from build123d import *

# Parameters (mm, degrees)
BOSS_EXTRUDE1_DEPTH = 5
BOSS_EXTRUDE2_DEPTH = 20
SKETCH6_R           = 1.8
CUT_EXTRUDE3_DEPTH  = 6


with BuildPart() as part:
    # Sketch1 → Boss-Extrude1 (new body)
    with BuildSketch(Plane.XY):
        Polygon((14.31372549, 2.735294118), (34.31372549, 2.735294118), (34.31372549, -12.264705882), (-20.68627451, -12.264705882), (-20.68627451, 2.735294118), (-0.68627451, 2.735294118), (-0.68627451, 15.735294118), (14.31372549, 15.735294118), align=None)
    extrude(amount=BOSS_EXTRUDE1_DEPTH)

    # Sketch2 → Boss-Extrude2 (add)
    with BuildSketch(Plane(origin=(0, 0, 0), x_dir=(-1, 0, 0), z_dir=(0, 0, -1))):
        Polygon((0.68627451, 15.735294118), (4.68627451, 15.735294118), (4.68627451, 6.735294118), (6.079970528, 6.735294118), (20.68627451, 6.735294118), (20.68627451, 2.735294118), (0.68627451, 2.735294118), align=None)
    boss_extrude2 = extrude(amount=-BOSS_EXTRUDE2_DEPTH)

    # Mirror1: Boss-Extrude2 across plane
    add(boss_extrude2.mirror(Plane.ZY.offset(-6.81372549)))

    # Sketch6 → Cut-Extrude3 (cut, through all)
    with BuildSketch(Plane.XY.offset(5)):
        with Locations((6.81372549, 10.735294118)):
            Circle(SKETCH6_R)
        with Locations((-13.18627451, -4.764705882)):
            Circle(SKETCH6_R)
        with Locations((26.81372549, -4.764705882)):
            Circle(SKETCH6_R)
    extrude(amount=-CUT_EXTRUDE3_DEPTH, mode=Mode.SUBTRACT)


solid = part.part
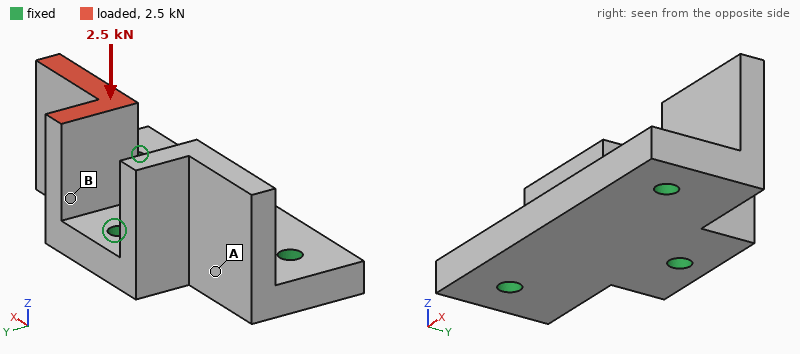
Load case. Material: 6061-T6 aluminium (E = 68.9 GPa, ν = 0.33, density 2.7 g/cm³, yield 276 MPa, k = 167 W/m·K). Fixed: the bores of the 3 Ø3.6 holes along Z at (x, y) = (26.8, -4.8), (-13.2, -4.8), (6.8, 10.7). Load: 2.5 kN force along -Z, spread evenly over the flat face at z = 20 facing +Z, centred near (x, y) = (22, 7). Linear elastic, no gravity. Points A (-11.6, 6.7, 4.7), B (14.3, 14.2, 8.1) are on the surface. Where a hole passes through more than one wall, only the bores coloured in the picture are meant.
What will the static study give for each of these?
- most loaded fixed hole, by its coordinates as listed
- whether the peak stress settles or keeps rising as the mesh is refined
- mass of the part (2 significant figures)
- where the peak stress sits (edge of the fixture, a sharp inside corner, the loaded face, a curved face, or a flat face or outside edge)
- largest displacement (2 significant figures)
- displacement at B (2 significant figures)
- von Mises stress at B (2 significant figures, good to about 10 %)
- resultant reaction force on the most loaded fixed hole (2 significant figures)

(26.8, -4.8)
keeps rising
26 g
edge of the fixture
75 µm
32 µm
54 MPa
1.4 kN
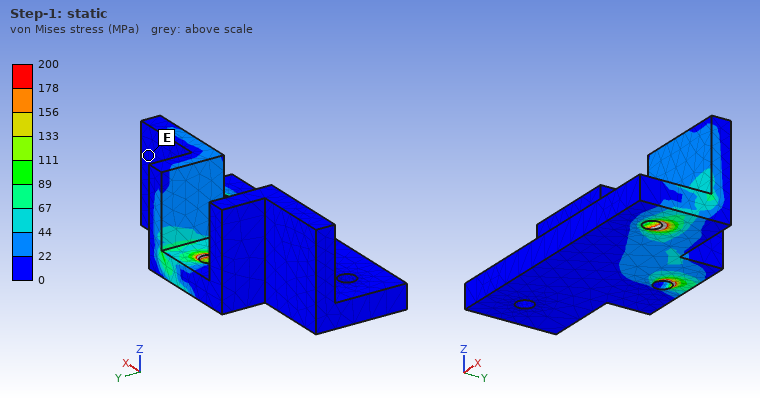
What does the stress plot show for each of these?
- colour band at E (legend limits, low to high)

0 to 22 MPa
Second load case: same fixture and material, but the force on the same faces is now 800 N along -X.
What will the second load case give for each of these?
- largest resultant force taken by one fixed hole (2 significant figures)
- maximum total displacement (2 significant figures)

610 N
65 µm
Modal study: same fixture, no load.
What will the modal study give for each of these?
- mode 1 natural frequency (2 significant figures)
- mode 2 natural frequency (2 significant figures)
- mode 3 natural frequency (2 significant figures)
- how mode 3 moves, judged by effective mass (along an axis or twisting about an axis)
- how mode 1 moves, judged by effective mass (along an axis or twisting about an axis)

9700 Hz
10 kHz
17 kHz
along X
along Y
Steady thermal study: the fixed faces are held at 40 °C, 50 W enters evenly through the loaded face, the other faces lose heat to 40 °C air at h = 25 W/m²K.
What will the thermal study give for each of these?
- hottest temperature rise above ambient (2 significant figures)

58 K
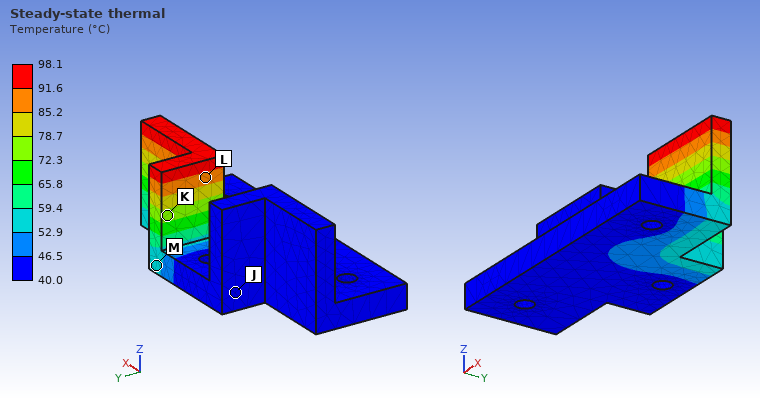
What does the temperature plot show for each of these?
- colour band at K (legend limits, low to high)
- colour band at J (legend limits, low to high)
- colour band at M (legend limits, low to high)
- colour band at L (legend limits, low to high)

72.3 to 78.7 °C
40.0 to 46.5 °C
52.9 to 59.4 °C
85.2 to 91.6 °C
